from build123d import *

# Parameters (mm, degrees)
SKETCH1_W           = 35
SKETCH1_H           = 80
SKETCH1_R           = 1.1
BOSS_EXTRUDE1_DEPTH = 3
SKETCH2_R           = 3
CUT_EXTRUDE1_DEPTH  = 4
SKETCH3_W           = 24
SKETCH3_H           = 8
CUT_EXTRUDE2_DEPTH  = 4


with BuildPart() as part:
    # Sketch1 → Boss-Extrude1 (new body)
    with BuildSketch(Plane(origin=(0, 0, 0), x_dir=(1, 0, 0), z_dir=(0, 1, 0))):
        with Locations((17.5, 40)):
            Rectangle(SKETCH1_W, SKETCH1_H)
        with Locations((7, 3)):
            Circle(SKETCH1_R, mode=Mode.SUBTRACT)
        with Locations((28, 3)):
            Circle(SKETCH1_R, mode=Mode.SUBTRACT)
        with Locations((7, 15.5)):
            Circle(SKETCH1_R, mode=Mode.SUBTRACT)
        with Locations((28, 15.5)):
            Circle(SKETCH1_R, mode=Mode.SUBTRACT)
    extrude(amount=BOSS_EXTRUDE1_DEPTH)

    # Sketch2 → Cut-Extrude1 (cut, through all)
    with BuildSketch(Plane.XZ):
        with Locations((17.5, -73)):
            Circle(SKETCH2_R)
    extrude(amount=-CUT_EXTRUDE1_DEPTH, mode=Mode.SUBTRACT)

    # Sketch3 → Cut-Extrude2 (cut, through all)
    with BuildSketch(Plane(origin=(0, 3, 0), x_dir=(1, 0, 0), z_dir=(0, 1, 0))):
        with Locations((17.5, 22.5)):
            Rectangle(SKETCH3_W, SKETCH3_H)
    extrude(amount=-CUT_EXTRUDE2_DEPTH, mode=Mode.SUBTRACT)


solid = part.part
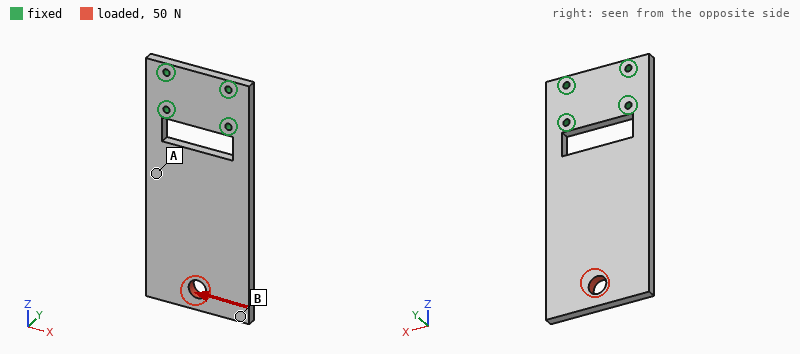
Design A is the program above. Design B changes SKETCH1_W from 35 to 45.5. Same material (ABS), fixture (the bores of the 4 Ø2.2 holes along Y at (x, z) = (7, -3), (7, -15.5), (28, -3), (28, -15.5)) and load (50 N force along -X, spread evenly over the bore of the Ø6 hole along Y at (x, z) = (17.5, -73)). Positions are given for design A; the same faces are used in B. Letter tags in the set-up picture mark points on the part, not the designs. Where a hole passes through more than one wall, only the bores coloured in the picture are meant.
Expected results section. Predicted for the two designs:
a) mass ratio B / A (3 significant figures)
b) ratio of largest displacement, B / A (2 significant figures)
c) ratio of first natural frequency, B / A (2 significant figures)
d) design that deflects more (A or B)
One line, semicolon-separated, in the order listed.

1.33; 0.56; 1.1; A
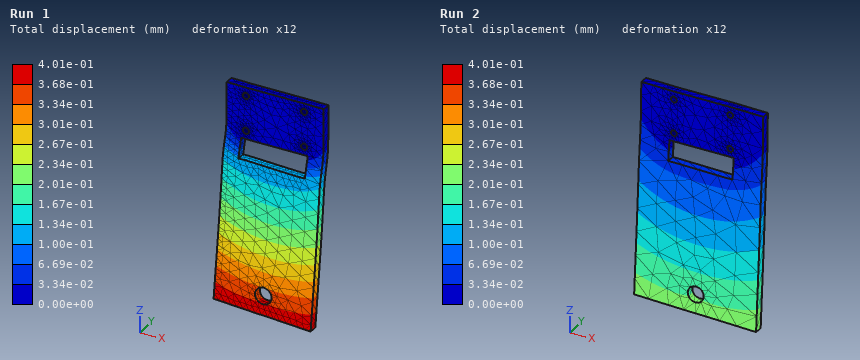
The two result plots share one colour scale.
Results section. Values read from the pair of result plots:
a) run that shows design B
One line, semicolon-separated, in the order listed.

Run 2
